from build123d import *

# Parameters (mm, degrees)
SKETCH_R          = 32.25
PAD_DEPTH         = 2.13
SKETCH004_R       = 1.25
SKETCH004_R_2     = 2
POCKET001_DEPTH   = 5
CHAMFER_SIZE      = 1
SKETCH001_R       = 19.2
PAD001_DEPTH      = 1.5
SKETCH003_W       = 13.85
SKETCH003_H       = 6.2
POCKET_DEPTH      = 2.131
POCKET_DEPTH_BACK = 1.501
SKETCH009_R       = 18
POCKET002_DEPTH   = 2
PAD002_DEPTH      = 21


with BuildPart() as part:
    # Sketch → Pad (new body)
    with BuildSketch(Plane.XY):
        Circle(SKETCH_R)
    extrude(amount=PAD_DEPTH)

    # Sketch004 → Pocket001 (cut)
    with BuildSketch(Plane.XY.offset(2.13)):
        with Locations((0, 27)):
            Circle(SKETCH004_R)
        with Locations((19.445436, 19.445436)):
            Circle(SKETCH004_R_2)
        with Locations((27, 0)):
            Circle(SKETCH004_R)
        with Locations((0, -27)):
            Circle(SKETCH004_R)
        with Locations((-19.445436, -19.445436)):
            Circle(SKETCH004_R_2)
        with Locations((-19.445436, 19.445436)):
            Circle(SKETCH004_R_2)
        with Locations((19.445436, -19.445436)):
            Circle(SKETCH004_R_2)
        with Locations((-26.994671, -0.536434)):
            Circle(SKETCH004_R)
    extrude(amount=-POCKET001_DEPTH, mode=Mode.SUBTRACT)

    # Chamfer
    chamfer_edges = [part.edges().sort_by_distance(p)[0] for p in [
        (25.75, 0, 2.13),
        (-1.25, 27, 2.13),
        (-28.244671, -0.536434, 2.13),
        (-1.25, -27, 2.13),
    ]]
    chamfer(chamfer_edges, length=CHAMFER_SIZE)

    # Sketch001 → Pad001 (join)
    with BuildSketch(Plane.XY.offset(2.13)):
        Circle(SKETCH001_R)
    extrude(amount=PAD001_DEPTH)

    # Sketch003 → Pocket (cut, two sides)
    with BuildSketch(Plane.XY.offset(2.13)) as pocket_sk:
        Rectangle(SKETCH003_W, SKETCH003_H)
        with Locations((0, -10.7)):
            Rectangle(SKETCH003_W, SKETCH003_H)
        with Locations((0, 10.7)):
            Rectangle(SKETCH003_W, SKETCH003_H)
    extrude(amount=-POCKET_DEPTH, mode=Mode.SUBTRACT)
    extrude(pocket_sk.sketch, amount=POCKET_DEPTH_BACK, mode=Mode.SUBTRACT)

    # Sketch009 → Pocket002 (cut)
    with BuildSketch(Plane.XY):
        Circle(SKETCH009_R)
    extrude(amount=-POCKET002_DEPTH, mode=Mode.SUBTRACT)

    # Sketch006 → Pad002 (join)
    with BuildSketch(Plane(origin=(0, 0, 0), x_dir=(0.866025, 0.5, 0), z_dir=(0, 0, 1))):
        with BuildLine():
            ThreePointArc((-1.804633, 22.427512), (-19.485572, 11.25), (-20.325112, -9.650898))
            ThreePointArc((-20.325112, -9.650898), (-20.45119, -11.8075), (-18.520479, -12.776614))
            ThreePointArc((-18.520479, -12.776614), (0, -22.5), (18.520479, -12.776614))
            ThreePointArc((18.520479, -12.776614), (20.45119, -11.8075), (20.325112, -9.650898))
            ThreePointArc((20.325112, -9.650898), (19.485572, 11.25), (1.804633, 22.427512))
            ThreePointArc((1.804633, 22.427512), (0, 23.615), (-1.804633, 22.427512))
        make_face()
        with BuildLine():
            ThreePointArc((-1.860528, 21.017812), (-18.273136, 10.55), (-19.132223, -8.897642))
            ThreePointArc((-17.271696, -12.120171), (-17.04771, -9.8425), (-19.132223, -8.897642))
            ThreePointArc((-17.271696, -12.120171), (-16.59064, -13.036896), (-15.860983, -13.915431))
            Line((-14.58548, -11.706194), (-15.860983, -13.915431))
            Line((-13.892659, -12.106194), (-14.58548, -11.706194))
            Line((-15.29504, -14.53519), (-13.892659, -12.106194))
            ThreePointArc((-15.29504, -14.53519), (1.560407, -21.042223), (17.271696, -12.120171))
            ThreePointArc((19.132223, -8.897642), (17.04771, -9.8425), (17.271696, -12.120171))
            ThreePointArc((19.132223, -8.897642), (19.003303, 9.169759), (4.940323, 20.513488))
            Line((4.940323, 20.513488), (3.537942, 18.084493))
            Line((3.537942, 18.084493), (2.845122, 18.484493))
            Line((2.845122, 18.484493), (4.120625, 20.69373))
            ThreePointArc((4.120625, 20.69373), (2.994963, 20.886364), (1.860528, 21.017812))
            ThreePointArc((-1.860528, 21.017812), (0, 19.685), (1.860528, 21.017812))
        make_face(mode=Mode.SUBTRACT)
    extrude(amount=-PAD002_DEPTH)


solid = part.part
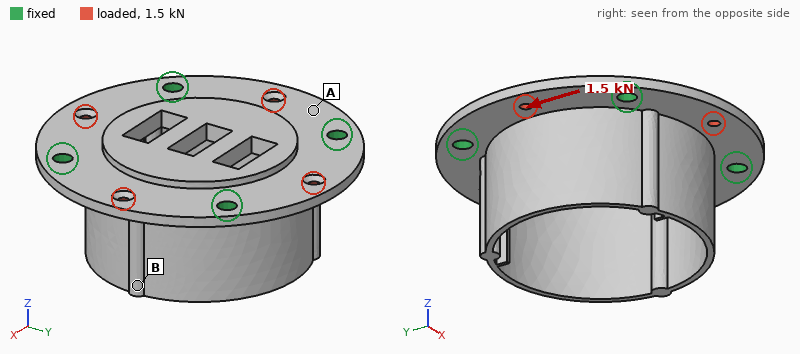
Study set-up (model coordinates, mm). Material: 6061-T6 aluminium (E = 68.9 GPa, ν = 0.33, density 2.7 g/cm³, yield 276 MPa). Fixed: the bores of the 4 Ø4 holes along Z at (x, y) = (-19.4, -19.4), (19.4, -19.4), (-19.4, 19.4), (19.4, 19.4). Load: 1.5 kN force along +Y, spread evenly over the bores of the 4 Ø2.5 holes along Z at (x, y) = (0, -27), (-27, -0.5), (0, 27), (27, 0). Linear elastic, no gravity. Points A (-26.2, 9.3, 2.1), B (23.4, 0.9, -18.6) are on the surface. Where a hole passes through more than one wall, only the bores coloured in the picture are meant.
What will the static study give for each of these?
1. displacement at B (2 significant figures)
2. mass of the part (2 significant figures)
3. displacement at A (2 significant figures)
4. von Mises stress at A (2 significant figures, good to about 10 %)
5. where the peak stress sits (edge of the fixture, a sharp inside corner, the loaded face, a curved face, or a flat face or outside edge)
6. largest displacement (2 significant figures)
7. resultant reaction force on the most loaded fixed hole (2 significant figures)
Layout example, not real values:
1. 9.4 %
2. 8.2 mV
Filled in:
1. 1.9 µm
2. 33 g
3. 2.2 µm
4. 8.7 MPa
5. the loaded face
6. 11 µm
7. 390 N
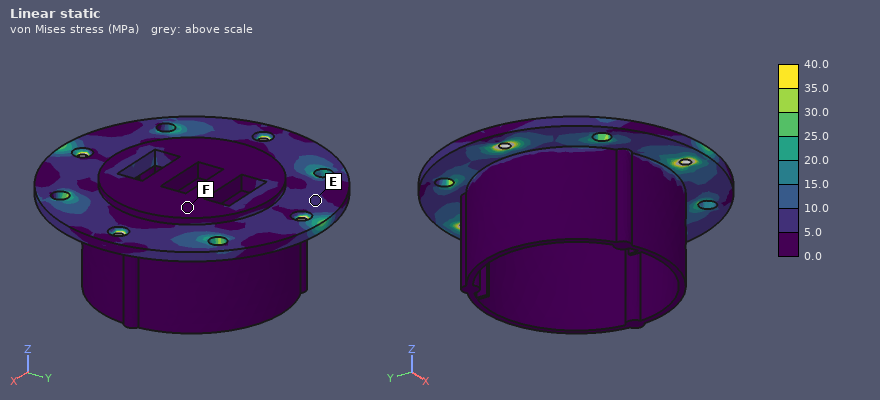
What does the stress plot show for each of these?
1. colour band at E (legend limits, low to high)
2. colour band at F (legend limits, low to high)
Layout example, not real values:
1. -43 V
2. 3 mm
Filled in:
1. 5.0 to 10.0 MPa
2. 0.0 to 5.0 MPa
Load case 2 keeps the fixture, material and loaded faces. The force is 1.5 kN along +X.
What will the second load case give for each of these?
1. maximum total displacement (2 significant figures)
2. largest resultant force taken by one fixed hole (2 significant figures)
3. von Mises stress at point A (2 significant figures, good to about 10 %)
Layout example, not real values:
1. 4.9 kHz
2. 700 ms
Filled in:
1. 10 µm
2. 390 N
3. 5.3 MPa
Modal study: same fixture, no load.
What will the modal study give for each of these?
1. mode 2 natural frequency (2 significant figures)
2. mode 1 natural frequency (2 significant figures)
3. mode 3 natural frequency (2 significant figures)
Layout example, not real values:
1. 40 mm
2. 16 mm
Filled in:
1. 6700 Hz
2. 4600 Hz
3. 7100 Hz
